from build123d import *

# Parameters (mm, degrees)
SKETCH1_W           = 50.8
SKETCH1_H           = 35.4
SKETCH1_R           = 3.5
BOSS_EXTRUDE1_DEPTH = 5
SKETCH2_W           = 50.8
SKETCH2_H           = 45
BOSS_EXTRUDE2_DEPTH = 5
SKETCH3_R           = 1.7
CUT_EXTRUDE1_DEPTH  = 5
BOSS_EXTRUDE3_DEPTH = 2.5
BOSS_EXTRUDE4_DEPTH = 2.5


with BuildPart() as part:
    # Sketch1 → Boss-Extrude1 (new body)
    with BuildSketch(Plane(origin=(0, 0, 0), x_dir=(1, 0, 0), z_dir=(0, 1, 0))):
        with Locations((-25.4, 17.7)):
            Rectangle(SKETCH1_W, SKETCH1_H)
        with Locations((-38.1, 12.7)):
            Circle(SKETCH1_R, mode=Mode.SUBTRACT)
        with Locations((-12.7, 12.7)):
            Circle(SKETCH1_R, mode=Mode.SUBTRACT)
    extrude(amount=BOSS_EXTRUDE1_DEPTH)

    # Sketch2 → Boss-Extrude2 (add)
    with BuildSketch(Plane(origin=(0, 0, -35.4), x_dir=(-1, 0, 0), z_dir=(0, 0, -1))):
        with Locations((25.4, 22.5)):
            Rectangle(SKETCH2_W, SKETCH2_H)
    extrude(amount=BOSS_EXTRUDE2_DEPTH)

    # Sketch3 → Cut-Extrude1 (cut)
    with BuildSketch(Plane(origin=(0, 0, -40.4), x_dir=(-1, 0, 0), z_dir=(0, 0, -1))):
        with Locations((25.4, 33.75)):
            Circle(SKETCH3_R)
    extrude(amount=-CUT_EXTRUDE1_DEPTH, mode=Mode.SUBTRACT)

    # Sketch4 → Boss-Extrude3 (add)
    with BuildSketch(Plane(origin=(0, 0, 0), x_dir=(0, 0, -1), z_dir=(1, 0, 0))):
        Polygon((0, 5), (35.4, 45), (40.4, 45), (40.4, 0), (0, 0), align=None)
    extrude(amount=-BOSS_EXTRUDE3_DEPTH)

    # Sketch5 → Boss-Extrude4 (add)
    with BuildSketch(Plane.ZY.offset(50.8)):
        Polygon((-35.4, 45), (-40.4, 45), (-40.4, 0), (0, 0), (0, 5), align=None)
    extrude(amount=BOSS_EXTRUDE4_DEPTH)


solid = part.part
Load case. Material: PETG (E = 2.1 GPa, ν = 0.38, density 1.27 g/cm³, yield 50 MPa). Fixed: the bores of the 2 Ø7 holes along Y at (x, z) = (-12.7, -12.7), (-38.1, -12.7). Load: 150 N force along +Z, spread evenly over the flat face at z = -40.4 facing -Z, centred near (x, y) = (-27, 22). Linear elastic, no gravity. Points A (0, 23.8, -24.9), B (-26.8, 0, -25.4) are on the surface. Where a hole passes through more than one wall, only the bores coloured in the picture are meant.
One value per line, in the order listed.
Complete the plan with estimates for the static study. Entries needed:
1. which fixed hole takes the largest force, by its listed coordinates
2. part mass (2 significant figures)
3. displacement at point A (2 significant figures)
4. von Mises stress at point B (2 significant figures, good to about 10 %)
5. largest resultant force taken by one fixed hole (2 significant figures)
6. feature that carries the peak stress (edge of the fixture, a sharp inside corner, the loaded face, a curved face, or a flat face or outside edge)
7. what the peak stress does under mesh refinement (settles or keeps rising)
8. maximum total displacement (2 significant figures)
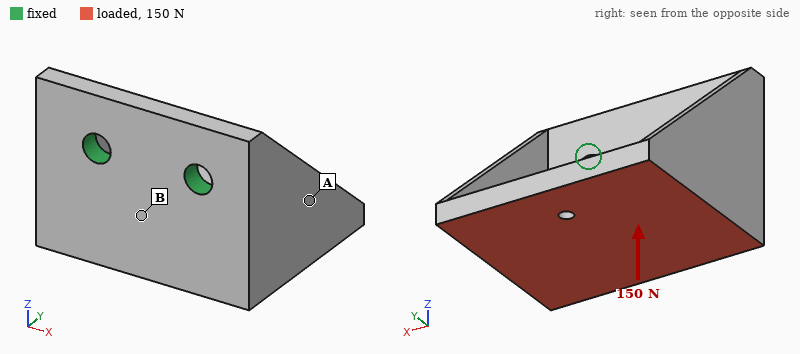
(-38.1, -12.7)
31 g
0.31 mm
3.5 MPa
82 N
edge of the fixture
keeps rising
0.89 mm
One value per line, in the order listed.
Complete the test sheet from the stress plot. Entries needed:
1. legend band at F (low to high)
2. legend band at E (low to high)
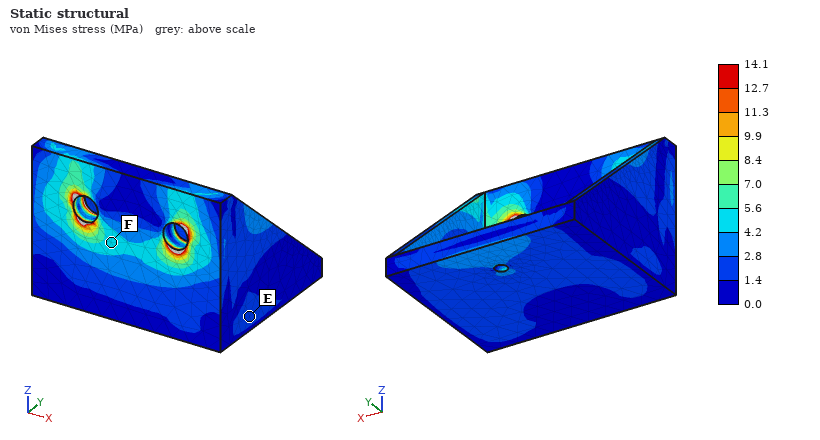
4.2 to 5.6 MPa
1.4 to 2.8 MPa
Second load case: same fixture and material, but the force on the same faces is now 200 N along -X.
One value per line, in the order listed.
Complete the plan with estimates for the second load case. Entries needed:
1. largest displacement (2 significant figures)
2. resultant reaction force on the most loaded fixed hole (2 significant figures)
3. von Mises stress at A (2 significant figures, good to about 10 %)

0.86 mm
230 N
2.0 MPa
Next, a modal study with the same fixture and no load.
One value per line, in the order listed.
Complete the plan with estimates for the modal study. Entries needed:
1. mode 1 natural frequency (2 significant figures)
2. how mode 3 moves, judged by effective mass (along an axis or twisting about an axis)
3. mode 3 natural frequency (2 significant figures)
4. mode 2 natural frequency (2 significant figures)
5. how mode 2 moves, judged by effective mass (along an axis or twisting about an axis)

520 Hz
along Y
1500 Hz
600 Hz
along X
